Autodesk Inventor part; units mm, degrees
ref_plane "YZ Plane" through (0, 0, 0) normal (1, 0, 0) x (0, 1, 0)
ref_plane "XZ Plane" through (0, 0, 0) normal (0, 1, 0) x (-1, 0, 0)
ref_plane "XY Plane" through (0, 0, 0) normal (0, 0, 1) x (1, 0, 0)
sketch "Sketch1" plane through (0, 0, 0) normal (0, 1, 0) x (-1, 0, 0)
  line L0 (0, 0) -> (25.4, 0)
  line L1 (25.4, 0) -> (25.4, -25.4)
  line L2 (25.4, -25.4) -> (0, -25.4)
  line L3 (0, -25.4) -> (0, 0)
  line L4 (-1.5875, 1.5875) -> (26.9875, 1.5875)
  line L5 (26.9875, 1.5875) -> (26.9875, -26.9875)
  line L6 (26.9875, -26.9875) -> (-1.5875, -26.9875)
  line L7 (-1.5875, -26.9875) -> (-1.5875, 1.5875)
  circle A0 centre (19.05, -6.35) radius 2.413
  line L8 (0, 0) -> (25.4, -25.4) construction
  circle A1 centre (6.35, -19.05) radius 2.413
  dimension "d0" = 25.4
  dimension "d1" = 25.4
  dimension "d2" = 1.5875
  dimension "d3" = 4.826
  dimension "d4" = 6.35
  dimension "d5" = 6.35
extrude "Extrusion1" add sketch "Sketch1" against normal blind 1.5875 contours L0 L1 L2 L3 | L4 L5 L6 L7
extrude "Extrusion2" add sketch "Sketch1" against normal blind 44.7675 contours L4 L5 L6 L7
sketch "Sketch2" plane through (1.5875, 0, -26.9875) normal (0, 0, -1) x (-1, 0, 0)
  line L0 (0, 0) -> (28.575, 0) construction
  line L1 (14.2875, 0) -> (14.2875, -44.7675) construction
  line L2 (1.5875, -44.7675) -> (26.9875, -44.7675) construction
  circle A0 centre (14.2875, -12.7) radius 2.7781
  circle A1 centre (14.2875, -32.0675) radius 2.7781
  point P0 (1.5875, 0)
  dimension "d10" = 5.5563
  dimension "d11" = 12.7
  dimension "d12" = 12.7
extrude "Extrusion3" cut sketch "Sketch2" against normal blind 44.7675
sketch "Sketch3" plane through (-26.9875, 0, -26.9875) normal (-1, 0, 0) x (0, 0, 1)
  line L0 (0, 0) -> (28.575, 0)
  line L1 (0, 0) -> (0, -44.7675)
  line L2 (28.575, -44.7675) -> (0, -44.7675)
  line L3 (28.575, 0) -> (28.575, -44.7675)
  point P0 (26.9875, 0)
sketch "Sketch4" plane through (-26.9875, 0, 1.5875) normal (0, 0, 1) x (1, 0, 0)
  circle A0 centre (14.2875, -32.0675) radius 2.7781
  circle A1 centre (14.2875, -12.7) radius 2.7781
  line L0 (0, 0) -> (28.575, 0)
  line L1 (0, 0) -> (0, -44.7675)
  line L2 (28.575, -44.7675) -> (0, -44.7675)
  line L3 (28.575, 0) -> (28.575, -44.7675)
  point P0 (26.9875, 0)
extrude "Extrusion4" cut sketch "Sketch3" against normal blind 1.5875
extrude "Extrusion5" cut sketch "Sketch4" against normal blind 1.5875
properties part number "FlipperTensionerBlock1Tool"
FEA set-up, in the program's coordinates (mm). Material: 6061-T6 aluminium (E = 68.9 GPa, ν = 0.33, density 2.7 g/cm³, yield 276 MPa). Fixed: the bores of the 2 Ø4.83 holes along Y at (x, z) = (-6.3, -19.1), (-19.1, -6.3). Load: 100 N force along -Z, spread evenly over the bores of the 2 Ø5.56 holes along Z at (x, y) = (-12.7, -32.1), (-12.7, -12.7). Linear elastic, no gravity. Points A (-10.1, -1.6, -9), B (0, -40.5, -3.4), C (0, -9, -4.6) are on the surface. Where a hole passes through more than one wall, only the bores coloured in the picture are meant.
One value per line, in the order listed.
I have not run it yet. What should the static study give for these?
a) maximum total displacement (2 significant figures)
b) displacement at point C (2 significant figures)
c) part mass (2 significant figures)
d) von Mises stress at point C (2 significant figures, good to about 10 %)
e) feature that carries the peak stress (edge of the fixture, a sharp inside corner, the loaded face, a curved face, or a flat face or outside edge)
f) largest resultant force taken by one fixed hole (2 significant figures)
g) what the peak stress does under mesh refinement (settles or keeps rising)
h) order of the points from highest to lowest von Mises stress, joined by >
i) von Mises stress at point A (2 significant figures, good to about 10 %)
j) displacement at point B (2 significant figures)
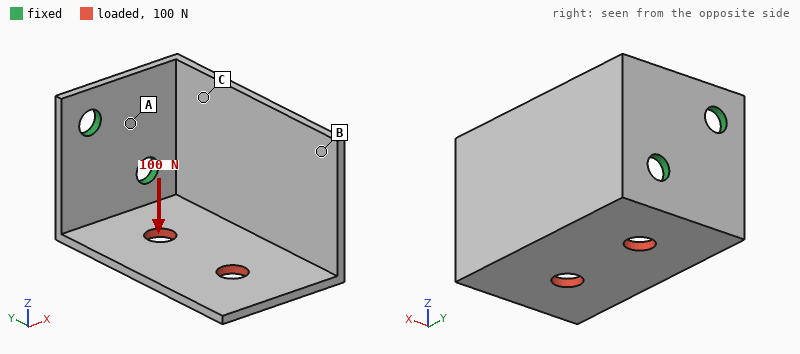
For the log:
0.64 mm
0.12 mm
12 g
24 MPa
edge of the fixture
67 N
keeps rising
A > C > B
44 MPa
0.35 mm
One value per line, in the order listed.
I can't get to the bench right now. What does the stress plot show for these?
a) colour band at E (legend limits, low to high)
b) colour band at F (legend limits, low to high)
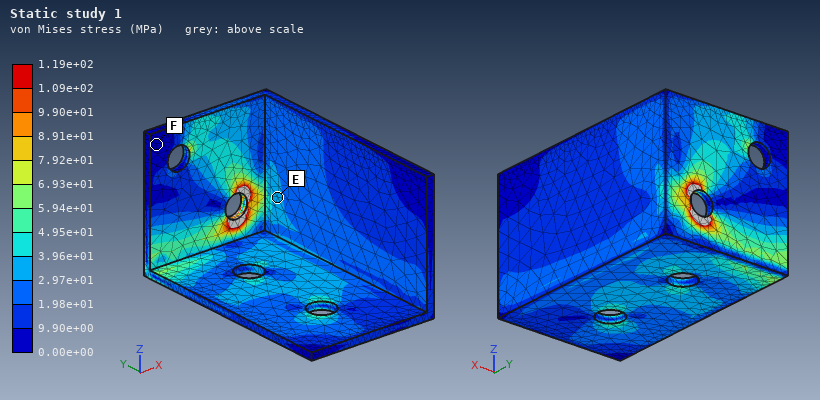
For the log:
2.97e+01 to 3.96e+01 MPa
0.00e+00 to 9.90e+00 MPa
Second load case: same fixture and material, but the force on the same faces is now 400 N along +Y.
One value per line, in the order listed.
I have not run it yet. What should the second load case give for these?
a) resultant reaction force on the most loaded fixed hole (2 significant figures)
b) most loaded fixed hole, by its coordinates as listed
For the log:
380 N
(-6.3, -19.1)
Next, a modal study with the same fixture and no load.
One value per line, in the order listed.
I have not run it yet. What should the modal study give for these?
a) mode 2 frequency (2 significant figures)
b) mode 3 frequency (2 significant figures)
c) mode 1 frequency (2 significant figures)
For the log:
1000 Hz
2200 Hz
970 Hz
